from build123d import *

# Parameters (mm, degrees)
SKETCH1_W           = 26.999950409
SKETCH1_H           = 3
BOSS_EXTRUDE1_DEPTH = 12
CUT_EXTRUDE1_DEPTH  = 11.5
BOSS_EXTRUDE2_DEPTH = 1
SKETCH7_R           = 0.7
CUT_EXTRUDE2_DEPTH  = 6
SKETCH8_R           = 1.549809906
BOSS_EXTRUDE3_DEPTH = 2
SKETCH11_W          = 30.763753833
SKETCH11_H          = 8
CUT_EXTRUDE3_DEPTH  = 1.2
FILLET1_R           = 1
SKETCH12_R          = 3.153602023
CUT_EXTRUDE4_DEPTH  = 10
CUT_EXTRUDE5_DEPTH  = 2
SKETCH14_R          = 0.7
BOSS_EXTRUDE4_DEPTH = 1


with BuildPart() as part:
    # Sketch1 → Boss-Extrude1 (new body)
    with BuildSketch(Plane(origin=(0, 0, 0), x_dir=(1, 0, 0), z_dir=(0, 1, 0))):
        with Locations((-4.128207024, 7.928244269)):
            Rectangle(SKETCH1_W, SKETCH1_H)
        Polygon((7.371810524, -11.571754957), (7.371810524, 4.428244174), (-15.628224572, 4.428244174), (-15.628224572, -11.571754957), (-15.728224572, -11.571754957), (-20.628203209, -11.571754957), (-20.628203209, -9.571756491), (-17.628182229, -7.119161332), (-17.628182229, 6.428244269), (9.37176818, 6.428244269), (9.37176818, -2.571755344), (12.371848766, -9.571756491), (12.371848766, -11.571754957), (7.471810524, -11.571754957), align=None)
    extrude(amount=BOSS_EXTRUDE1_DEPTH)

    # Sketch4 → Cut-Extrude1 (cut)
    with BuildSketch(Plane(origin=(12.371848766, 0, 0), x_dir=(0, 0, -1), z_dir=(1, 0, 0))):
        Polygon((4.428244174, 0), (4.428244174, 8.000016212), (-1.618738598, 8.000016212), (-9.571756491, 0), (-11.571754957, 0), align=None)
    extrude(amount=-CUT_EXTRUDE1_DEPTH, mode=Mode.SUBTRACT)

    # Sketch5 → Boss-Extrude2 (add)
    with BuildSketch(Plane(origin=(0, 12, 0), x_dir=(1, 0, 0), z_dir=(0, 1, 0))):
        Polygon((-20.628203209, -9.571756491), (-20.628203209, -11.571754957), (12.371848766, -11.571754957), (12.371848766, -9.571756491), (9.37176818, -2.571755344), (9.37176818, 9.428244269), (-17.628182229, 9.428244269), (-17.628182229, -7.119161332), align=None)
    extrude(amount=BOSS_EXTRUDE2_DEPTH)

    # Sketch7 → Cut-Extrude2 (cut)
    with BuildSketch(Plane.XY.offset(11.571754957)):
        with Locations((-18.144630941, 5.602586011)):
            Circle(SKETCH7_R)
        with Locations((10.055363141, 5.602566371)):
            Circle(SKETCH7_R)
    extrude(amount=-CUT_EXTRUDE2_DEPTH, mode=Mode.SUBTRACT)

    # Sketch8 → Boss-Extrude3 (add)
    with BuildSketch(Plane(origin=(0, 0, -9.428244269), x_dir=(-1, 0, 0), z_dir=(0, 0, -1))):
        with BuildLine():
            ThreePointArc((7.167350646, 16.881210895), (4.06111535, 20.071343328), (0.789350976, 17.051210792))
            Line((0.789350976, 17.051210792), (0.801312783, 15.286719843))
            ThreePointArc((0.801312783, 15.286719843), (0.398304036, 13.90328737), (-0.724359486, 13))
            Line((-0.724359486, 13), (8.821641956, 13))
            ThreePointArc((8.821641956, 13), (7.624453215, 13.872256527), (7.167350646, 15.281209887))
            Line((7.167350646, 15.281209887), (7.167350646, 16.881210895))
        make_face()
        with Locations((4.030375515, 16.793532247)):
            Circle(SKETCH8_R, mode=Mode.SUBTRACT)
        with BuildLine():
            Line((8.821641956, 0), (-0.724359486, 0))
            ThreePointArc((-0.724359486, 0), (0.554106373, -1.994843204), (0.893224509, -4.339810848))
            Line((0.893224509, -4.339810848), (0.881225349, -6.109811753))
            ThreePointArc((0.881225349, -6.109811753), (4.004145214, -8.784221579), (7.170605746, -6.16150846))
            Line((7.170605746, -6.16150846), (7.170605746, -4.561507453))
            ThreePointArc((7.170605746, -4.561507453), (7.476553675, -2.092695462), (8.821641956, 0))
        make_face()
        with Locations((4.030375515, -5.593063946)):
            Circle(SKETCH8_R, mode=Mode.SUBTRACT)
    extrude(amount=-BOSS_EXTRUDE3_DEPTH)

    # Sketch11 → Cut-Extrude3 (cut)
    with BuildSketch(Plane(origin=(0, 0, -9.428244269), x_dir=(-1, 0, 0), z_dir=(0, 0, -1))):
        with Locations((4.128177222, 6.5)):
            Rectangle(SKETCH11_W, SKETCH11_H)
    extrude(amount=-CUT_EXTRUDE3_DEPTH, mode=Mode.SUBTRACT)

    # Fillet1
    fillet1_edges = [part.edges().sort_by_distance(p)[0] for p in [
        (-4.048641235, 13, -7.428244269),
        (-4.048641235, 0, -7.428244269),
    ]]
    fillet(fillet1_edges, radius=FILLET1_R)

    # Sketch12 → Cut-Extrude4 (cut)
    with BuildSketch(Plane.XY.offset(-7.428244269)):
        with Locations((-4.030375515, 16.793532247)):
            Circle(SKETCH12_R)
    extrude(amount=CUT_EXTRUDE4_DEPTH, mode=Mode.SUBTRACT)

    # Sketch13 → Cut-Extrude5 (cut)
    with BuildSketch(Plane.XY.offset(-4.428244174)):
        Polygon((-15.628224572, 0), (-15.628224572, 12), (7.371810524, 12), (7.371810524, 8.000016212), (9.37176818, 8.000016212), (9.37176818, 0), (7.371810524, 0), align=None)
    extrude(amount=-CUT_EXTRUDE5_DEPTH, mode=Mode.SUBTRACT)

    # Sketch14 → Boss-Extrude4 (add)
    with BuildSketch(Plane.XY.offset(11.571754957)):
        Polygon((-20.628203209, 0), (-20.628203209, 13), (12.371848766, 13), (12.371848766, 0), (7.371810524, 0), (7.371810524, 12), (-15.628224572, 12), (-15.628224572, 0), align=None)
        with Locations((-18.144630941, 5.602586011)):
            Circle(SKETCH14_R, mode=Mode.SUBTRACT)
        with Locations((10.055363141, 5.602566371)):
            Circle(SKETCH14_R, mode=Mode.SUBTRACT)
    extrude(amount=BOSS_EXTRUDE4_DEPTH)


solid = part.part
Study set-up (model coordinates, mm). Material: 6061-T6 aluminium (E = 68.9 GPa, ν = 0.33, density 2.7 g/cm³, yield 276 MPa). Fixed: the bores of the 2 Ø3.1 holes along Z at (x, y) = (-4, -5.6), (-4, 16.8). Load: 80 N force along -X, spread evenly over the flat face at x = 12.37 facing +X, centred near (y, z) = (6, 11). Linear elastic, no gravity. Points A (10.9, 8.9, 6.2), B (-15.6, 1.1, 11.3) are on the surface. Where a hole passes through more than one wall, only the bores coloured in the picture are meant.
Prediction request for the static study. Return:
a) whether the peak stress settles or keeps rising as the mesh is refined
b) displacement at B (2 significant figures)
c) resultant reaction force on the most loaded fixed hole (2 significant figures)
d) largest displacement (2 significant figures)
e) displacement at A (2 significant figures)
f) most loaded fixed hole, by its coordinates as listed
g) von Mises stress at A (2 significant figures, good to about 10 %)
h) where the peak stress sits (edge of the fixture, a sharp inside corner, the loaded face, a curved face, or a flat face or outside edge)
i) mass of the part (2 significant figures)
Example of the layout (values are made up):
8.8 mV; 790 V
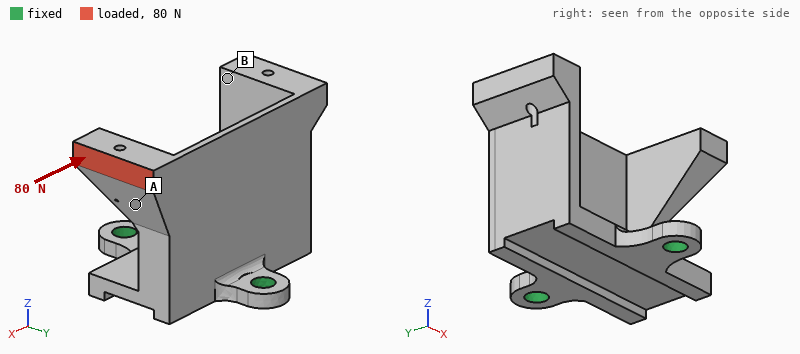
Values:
keeps rising; 0.14 mm; 42 N; 0.31 mm; 0.17 mm; (-4, 16.8); 30 MPa; edge of the fixture; 6.9 g
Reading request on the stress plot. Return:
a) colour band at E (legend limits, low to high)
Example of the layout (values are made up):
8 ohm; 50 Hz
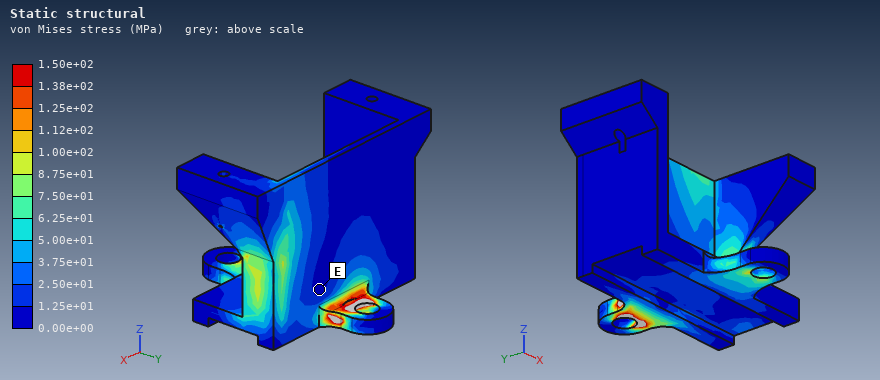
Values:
0.00e+00 to 1.25e+01 MPa
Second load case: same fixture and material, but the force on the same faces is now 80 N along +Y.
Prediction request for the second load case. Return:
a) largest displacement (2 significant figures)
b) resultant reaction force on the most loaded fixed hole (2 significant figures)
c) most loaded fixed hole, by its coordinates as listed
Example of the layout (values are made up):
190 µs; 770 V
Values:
0.40 mm; 210 N; (-4, -5.6)
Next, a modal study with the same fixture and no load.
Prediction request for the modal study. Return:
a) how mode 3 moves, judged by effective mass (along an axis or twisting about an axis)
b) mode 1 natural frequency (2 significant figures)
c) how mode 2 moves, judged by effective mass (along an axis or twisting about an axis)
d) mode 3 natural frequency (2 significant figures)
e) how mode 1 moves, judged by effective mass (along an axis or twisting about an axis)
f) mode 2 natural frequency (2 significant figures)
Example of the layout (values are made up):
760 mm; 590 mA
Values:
along Y; 1900 Hz; along Y; 3400 Hz; along X; 2500 Hz
